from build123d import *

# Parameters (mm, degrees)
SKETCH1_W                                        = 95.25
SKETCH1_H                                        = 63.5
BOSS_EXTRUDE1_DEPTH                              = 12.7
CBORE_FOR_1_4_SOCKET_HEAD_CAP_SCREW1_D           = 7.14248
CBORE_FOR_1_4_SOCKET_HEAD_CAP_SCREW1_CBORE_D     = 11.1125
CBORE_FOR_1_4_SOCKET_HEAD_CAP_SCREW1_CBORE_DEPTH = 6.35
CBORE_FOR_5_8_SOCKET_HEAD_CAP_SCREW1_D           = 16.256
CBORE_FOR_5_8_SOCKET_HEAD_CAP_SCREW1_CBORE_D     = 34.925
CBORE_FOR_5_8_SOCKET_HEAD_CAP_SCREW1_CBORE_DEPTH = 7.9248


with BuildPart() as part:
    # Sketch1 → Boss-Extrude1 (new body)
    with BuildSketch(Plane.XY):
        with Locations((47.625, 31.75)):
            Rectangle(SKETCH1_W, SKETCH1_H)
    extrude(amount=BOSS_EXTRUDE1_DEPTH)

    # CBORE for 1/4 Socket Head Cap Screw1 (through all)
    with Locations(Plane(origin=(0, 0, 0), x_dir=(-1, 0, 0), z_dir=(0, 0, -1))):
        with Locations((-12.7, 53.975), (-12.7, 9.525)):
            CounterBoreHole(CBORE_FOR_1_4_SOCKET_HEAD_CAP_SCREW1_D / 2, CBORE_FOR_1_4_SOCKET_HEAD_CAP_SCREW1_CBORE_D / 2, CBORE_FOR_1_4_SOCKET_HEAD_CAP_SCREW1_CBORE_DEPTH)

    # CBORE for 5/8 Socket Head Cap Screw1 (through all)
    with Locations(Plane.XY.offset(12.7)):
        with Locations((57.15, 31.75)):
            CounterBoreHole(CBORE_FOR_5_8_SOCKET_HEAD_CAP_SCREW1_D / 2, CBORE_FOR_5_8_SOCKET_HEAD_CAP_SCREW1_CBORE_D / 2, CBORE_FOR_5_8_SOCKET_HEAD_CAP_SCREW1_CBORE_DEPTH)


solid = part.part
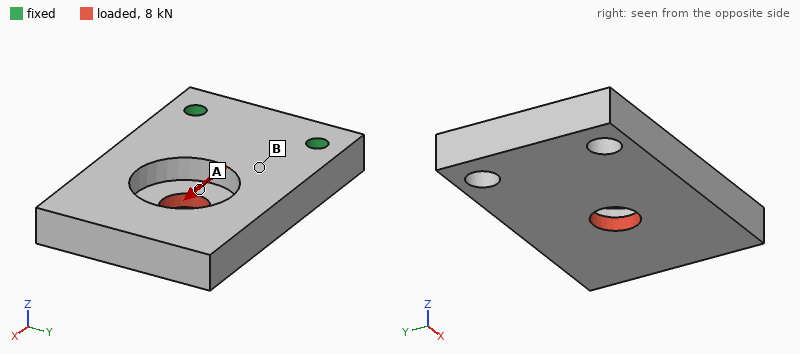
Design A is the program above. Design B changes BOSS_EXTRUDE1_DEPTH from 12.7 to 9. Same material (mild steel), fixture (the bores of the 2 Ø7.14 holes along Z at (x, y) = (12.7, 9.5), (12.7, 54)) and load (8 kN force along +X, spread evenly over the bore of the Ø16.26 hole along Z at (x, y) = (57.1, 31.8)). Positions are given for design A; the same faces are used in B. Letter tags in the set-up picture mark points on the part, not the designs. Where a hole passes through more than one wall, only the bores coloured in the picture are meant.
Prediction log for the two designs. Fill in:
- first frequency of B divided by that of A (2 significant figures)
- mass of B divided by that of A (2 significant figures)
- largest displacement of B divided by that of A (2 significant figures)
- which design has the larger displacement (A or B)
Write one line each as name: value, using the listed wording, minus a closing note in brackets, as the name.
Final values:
first frequency of B divided by that of A: 0.64
mass of B divided by that of A: 0.72
largest displacement of B divided by that of A: 2.4
which design has the larger displacement: B
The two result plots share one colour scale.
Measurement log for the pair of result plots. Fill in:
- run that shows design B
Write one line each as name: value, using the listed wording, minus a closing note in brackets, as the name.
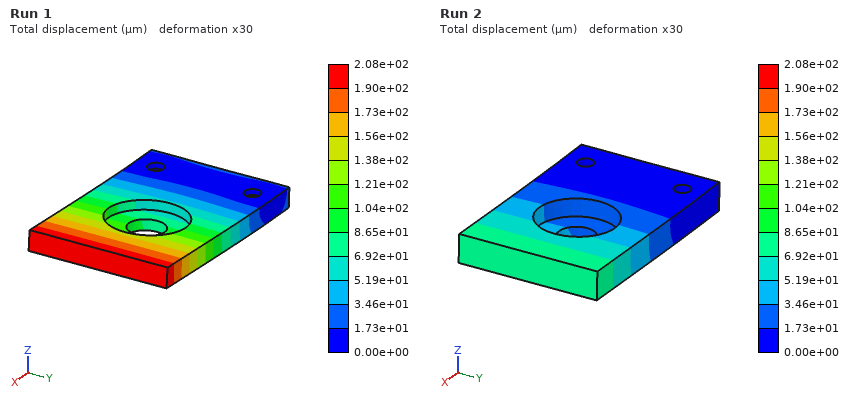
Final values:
run that shows design B: Run 1
